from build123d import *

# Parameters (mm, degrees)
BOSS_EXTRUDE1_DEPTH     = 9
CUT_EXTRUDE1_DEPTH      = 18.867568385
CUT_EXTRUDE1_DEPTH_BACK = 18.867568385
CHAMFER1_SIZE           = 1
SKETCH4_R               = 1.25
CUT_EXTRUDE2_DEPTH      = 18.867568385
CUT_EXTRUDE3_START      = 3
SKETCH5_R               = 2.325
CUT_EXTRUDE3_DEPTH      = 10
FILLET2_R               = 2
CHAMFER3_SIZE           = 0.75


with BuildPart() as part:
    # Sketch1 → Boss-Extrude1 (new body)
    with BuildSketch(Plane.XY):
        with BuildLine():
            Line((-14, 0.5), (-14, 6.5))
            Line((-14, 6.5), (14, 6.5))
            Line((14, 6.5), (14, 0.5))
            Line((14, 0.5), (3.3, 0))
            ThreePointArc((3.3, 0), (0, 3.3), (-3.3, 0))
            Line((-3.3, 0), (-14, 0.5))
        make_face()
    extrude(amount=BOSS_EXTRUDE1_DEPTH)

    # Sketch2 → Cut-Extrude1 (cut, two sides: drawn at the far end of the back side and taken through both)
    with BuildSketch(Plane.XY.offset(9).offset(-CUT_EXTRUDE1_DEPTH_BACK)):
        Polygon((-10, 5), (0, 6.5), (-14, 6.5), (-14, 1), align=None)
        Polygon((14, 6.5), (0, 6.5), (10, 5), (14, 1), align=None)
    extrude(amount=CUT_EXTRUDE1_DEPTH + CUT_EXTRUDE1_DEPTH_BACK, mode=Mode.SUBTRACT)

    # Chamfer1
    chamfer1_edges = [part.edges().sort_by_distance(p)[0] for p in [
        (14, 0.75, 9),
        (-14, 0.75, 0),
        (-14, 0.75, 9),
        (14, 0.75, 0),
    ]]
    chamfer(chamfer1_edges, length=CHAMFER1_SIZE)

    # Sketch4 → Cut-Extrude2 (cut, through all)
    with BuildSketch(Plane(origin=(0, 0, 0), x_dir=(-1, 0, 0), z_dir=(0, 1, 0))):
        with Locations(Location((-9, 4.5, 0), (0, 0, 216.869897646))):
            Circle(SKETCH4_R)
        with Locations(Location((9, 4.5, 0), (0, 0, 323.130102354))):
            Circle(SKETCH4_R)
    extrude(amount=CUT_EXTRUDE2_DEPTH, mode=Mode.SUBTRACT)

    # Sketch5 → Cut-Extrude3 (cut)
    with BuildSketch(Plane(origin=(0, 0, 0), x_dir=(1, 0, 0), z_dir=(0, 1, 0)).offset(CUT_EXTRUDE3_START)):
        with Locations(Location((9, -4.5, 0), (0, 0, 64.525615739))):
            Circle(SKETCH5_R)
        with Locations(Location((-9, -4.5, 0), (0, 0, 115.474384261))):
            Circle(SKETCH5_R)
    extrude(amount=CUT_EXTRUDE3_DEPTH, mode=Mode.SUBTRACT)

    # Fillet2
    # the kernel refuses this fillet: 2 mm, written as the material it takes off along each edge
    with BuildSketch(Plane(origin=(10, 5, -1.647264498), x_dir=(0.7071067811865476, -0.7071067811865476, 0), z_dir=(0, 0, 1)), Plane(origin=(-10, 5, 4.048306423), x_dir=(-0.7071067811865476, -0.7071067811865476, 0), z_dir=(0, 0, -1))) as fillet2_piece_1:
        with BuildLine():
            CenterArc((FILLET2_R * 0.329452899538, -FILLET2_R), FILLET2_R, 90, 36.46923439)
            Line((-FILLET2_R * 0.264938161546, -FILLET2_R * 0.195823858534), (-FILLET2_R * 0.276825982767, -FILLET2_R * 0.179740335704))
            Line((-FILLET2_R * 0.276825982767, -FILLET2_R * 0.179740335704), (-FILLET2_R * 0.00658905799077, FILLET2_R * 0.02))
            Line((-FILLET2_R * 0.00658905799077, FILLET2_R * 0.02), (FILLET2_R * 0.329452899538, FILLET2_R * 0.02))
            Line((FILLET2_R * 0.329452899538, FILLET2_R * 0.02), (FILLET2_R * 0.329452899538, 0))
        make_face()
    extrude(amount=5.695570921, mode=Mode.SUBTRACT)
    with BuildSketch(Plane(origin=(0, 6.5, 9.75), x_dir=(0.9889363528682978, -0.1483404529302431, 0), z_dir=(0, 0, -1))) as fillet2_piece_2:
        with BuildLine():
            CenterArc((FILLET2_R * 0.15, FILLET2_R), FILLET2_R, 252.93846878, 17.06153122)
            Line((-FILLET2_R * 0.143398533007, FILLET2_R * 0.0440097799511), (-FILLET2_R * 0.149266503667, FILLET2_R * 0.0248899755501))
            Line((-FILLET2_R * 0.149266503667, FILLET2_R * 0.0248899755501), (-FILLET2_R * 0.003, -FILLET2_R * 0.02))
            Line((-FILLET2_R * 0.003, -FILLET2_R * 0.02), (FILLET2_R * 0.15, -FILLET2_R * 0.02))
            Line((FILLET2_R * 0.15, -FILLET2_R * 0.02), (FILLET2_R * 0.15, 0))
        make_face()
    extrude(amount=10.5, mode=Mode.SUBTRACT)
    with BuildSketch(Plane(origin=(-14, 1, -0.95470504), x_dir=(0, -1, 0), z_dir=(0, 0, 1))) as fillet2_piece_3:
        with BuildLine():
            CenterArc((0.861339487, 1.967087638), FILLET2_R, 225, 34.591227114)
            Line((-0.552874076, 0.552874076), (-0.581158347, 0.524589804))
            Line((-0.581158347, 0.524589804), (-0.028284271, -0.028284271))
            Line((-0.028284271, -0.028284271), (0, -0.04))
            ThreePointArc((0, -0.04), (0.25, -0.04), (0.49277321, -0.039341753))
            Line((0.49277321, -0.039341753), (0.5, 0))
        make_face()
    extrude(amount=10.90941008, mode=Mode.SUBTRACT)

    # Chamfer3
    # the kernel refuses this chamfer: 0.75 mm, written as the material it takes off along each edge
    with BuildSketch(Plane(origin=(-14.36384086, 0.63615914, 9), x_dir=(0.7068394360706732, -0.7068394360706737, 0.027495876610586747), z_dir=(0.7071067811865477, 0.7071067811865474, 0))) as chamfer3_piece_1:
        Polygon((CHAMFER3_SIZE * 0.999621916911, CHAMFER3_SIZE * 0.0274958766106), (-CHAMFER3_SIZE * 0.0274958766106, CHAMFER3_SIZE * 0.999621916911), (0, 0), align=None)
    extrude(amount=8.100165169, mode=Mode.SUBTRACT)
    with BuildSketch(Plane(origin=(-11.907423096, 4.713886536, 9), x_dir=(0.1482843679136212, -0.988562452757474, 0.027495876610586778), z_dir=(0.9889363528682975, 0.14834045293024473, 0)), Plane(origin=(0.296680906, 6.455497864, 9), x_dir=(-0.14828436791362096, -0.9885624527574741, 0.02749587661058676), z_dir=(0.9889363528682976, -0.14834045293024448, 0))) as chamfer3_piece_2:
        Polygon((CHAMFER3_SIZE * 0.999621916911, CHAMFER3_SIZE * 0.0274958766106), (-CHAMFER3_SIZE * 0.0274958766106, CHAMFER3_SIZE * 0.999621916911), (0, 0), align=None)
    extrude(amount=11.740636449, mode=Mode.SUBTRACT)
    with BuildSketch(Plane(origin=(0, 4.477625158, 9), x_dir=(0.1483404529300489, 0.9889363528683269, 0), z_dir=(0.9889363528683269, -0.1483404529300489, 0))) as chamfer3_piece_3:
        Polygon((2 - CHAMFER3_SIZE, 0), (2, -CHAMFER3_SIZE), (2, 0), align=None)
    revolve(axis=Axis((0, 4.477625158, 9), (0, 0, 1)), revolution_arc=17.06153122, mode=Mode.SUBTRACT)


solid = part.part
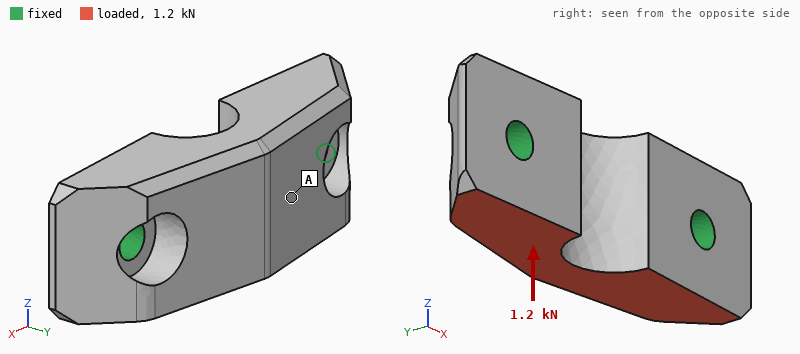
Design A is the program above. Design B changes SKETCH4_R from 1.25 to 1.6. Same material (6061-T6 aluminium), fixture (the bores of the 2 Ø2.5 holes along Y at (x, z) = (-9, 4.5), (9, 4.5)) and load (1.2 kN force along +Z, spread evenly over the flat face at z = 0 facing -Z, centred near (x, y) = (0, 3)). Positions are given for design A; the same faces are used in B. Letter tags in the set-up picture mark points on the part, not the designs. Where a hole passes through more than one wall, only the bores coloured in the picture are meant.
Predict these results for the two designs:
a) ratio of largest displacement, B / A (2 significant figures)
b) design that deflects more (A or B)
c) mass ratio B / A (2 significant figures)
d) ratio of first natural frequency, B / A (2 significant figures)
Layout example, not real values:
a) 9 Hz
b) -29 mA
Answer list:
a) 0.78
b) A
c) 0.98
d) 1.2
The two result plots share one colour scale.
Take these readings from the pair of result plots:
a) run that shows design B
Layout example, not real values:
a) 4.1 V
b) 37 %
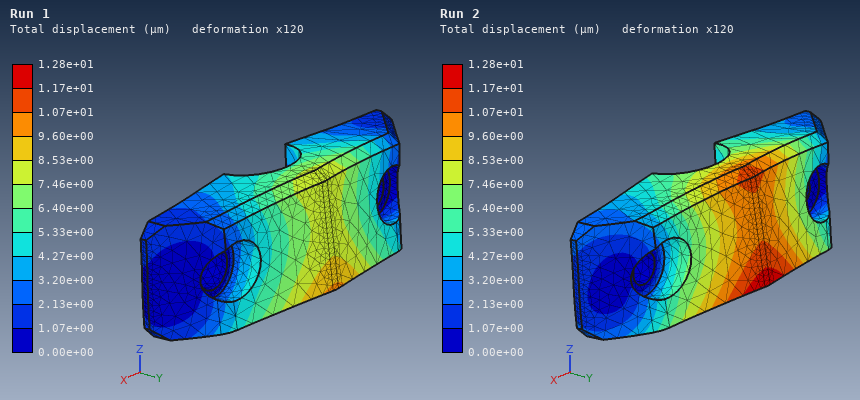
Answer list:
a) Run 1
